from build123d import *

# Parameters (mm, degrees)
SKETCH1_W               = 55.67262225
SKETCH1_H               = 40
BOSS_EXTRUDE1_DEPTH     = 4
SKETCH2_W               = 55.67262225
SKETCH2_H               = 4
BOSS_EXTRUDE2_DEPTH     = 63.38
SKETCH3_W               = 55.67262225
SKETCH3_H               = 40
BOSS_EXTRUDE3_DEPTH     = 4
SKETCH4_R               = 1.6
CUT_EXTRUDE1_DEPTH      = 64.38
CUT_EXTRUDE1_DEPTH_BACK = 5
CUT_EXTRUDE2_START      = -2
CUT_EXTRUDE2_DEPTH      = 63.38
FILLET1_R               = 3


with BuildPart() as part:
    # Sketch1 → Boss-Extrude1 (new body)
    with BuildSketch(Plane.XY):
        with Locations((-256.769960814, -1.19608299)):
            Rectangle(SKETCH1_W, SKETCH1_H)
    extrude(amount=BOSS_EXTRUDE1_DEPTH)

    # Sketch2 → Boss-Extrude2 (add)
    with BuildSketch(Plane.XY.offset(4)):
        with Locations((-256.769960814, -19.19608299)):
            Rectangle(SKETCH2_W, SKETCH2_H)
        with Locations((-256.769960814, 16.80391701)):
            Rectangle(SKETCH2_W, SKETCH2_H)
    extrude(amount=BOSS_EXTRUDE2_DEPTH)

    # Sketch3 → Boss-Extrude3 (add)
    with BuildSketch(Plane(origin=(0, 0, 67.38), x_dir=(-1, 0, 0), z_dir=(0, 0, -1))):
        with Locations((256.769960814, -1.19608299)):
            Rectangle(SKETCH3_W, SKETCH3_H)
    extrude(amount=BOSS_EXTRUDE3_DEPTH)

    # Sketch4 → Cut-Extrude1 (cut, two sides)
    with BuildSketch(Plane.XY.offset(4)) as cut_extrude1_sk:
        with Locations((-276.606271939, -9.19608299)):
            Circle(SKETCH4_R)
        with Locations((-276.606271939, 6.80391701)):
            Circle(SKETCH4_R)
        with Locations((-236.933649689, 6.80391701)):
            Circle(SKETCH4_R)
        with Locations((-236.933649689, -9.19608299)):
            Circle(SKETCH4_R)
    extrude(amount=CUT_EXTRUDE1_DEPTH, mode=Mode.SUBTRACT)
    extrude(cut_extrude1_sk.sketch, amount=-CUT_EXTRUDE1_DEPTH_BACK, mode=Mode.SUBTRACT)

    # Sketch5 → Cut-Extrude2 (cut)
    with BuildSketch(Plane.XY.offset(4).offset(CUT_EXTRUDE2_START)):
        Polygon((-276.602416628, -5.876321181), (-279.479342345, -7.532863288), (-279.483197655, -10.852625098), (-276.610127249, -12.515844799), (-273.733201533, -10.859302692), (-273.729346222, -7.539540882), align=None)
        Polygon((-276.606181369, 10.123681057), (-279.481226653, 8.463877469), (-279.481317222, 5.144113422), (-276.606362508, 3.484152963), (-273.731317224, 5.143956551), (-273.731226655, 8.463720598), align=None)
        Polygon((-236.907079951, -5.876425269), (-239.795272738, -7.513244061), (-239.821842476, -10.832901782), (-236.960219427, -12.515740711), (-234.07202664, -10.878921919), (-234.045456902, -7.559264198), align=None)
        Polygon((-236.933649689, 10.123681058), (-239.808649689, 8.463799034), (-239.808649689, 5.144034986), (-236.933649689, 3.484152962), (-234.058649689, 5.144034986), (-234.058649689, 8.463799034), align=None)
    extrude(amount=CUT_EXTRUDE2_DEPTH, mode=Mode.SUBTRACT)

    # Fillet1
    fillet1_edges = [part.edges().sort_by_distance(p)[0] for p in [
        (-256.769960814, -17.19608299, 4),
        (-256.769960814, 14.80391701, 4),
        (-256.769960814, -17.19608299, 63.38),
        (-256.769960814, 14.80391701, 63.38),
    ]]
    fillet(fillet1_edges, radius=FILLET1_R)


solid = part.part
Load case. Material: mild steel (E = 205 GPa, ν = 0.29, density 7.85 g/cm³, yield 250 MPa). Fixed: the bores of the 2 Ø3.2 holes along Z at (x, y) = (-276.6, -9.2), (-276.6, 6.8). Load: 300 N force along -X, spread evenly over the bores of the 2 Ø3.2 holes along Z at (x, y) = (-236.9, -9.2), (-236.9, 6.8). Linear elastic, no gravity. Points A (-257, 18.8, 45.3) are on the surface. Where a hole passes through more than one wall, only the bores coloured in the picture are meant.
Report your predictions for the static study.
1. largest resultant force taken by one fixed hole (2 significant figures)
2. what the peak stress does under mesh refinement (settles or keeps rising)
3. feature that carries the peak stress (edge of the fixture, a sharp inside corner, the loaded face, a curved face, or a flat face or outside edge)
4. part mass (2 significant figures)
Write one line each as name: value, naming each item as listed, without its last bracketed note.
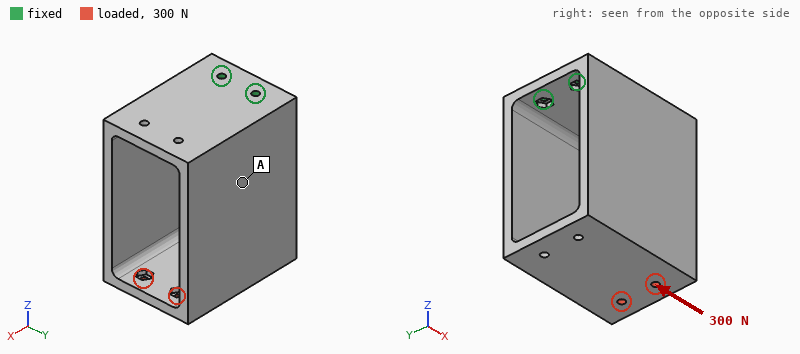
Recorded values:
largest resultant force taken by one fixed hole: 320 N
what the peak stress does under mesh refinement: keeps rising
feature that carries the peak stress: edge of the fixture
part mass: 350 g
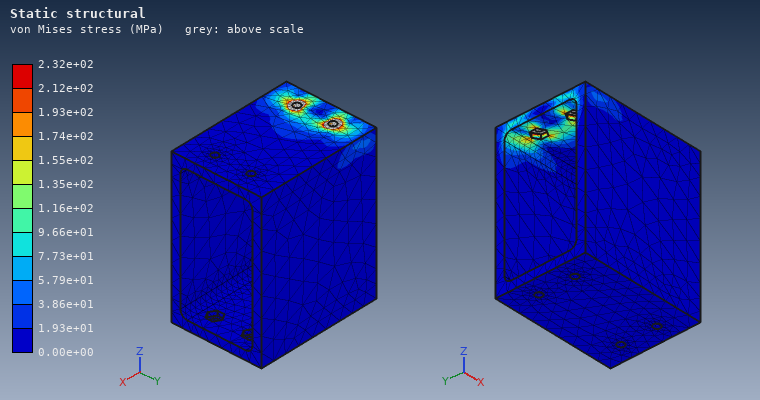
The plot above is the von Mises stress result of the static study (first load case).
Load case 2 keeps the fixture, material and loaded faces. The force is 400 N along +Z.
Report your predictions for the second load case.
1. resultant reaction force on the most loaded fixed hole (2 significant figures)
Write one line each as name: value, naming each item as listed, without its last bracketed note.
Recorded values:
resultant reaction force on the most loaded fixed hole: 210 N
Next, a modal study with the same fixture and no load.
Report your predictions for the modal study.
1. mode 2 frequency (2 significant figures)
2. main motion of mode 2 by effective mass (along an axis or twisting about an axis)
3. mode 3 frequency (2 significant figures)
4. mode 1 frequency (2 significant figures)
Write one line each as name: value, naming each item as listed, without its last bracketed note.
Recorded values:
mode 2 frequency: 560 Hz
main motion of mode 2 by effective mass: along Y
mode 3 frequency: 1700 Hz
mode 1 frequency: 340 Hz
